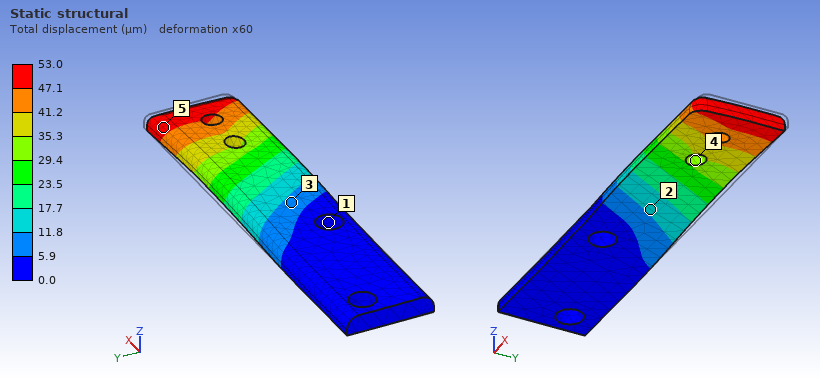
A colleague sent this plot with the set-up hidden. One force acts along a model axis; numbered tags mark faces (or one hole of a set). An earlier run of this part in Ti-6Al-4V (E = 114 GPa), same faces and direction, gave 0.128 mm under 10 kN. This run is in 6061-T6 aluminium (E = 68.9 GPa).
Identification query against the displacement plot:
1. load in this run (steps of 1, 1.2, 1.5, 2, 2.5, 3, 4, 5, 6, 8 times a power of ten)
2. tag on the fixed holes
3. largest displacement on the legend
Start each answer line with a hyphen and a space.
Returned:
- 2.5 kN
- 1
- 53.0 µm
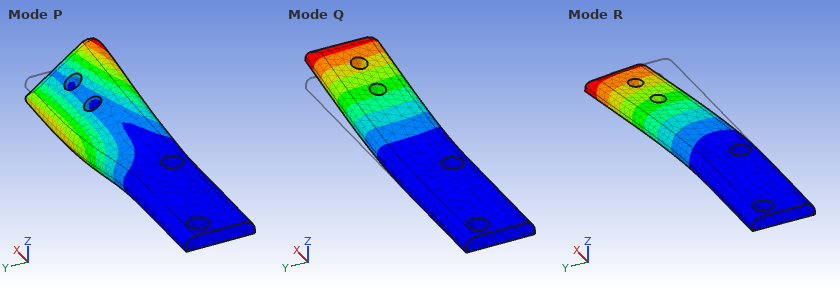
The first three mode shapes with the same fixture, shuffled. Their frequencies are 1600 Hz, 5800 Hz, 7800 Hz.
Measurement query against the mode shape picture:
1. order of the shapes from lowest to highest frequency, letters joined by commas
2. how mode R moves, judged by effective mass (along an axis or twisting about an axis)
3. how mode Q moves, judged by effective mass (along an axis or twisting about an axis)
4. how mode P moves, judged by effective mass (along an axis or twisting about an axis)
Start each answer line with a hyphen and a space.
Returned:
- Q, R, P
- along Y
- along Z
- twisting about X
